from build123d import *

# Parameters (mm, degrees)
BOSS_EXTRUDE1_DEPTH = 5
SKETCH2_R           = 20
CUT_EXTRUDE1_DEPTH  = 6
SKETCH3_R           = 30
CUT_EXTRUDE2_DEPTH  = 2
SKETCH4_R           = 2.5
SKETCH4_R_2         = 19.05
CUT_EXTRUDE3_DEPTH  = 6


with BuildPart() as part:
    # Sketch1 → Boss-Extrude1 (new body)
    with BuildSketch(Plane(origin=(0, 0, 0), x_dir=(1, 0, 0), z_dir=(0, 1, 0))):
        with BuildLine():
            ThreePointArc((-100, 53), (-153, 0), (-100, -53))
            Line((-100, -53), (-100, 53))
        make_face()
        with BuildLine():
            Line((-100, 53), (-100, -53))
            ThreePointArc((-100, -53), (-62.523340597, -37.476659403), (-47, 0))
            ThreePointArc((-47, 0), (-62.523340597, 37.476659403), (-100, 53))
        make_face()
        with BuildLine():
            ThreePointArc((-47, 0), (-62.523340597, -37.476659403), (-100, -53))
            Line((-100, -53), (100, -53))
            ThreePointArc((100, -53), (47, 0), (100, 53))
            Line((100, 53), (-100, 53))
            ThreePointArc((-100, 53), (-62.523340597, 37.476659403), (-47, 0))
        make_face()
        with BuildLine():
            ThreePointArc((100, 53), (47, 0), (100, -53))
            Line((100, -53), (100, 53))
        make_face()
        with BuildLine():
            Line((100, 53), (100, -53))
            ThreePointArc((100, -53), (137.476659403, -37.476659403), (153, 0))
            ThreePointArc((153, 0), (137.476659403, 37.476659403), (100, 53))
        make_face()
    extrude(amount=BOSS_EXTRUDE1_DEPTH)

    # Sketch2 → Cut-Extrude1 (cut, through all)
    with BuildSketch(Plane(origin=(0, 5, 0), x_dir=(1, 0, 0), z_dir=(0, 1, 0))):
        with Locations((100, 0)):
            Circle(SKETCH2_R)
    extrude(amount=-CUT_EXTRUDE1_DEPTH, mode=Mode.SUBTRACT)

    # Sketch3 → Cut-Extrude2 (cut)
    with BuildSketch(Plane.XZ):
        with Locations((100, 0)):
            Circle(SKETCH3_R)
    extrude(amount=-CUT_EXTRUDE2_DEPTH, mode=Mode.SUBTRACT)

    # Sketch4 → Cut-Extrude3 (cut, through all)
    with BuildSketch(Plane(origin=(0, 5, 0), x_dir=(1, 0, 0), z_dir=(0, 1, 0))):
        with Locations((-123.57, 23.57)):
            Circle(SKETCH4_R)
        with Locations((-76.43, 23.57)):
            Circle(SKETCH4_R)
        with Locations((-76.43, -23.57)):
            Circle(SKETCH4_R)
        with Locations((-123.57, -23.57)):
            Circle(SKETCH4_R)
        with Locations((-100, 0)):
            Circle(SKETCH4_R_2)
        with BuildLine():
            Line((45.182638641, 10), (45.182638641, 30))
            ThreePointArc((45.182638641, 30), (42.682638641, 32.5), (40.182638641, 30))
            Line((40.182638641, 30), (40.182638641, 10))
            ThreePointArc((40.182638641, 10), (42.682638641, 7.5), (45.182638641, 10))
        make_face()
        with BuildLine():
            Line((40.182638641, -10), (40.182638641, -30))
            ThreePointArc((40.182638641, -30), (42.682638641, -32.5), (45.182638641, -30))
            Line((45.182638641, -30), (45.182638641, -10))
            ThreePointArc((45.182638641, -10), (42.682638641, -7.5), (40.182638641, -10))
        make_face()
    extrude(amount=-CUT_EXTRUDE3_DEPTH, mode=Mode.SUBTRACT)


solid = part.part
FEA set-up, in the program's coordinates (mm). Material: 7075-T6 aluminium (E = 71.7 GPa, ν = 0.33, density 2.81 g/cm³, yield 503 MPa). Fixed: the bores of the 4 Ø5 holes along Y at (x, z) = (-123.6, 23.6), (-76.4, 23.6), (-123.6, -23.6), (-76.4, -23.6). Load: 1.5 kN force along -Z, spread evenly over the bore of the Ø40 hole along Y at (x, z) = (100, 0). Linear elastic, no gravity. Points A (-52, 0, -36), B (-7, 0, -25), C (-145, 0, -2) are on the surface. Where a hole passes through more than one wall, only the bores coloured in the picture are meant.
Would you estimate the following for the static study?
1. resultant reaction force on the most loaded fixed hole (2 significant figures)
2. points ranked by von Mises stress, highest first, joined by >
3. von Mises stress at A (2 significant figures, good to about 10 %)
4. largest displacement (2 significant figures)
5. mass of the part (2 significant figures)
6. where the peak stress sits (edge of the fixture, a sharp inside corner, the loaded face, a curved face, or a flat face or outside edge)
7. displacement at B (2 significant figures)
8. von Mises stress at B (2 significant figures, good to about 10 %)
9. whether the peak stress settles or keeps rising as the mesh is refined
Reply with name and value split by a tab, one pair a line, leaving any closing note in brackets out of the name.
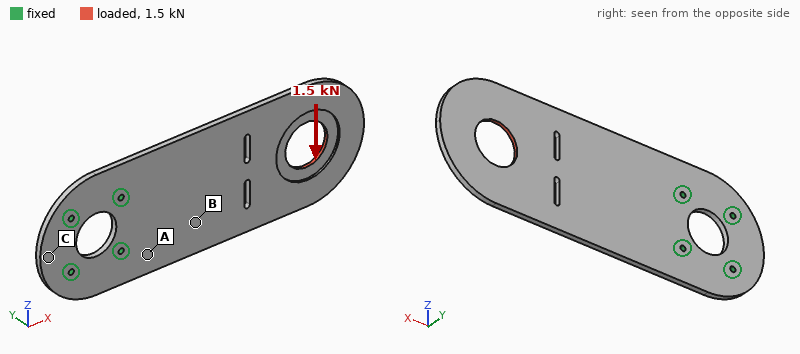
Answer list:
resultant reaction force on the most loaded fixed hole	3.3 kN
points ranked by von Mises stress, highest first, joined by >	A > B > C
von Mises stress at A	18 MPa
largest displacement	0.20 mm
mass of the part	370 g
where the peak stress sits	edge of the fixture
displacement at B	0.045 mm
von Mises stress at B	8.4 MPa
whether the peak stress settles or keeps rising as the mesh is refined	keeps rising
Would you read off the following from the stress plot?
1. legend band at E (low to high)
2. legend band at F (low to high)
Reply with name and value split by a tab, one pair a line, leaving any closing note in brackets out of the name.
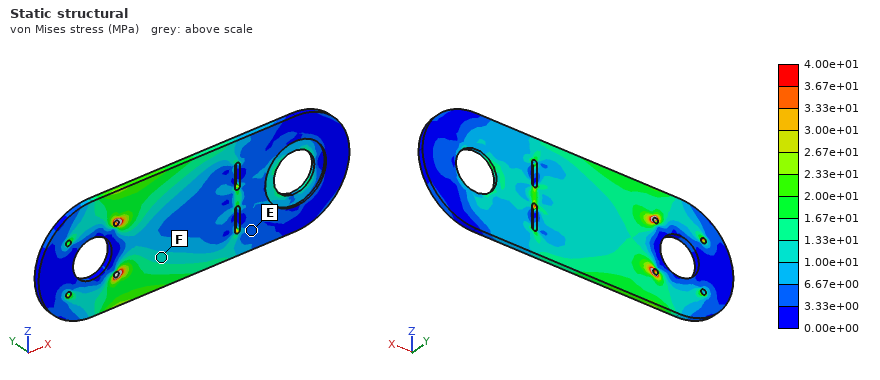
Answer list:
legend band at E	3.33e+00 to 6.67e+00 MPa
legend band at F	1.00e+01 to 1.33e+01 MPa
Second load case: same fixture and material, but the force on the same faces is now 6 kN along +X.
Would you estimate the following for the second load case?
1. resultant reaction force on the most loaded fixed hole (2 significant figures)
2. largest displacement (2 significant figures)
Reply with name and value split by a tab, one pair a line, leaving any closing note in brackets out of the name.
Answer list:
resultant reaction force on the most loaded fixed hole	2.5 kN
largest displacement	2.0 mm
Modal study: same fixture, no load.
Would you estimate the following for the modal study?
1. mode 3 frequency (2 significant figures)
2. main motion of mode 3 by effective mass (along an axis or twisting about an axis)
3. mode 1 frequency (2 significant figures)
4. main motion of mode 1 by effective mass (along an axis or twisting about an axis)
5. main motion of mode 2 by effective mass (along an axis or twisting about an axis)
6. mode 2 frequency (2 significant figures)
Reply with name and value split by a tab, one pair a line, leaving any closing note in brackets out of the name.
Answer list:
mode 3 frequency	470 Hz
main motion of mode 3 by effective mass	along Y
mode 1 frequency	92 Hz
main motion of mode 1 by effective mass	along Y
main motion of mode 2 by effective mass	twisting about X
mode 2 frequency	380 Hz
